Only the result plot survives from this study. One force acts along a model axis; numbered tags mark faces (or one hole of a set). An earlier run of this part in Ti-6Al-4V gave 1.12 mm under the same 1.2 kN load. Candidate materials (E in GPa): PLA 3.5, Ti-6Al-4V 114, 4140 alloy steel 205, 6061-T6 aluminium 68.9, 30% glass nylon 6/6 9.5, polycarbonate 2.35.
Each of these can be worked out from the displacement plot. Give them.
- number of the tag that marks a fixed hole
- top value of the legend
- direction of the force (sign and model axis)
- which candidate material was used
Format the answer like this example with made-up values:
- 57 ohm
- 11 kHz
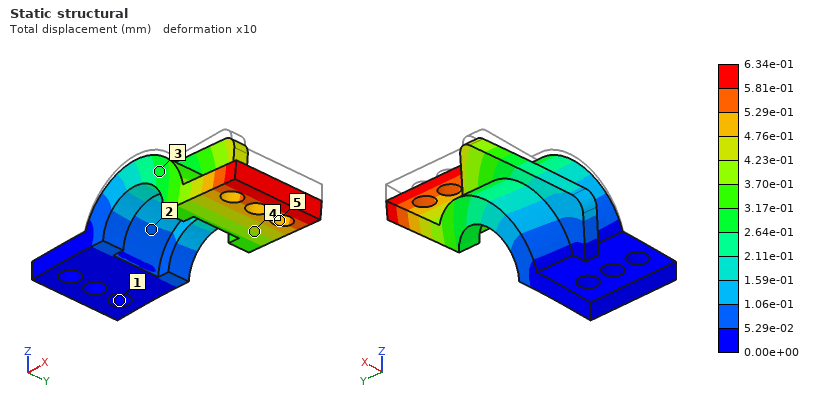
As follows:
- 1
- 6.34e-01 mm
- -Z
- 4140 alloy steel
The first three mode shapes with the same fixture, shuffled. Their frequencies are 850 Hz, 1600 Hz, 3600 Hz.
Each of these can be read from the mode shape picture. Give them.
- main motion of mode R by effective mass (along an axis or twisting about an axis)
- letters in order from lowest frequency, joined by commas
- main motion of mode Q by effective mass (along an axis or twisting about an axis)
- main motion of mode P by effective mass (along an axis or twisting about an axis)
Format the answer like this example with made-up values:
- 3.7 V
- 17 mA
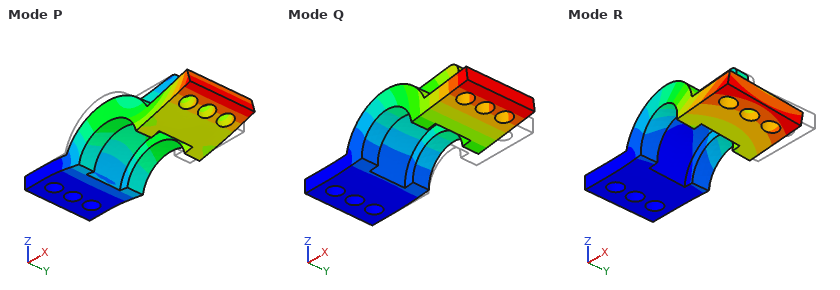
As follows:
- along Y
- Q, R, P
- along Z
- along X
